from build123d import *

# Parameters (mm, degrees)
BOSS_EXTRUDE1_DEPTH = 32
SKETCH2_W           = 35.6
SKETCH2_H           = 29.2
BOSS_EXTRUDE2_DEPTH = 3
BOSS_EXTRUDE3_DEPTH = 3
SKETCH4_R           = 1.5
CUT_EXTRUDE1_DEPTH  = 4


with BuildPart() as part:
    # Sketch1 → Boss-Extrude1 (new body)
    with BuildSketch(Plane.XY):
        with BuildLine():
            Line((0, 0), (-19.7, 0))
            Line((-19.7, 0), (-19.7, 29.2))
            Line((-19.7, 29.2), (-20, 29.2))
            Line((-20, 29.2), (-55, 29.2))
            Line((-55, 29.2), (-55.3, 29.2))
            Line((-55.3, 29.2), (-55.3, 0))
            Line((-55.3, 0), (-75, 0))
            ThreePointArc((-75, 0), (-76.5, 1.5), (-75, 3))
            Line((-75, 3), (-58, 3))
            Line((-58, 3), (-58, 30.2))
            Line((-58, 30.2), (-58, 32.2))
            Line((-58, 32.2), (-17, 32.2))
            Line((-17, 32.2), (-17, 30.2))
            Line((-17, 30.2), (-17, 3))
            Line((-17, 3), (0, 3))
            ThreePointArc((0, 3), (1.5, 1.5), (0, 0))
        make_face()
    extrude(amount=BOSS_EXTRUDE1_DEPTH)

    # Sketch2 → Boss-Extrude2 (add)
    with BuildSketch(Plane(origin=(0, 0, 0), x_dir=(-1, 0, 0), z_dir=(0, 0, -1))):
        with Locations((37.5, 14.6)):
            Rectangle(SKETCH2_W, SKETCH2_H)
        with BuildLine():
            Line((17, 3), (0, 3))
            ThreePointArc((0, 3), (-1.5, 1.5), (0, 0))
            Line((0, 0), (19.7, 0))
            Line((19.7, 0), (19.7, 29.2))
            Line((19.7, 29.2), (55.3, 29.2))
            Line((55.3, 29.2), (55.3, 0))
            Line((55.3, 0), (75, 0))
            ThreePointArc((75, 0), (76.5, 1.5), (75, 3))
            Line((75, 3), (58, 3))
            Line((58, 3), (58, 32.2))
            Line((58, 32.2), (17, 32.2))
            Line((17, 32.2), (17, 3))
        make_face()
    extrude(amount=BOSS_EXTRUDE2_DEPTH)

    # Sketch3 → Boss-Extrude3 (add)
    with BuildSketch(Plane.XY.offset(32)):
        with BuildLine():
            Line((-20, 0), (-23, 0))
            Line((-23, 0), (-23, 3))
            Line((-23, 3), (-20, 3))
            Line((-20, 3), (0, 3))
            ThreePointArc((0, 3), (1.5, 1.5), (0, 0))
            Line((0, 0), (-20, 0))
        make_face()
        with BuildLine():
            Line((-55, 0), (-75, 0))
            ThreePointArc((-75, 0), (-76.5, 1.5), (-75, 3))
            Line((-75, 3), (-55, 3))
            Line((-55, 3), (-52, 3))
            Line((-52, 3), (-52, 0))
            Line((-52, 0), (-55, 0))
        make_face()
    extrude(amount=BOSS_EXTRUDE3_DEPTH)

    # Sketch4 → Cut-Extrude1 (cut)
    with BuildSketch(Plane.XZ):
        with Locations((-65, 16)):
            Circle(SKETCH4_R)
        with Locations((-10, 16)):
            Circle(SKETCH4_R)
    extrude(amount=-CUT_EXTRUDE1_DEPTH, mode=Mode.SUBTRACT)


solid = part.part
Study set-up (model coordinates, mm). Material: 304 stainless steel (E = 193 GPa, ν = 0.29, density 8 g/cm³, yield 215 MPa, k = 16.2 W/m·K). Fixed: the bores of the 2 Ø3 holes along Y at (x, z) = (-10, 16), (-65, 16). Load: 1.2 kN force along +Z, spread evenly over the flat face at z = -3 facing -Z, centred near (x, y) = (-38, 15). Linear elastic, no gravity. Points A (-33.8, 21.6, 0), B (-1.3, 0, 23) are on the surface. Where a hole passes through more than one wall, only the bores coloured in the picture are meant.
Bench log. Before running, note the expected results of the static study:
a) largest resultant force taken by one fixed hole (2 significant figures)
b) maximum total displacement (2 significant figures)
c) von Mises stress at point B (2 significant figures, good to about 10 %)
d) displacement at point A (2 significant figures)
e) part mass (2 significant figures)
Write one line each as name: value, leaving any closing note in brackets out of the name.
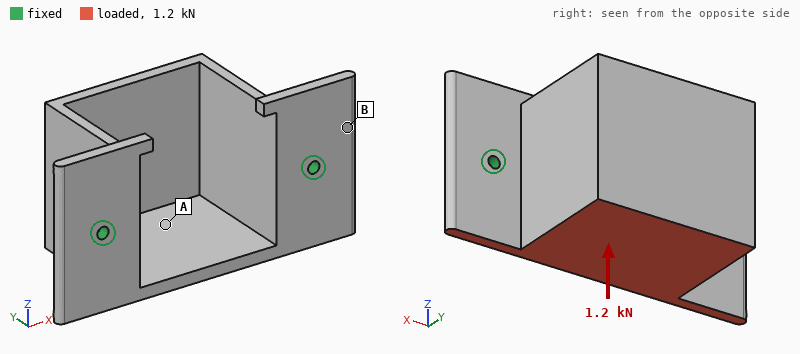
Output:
largest resultant force taken by one fixed hole: 670 N
maximum total displacement: 0.13 mm
von Mises stress at point B: 59 MPa
displacement at point A: 0.100 mm
part mass: 140 g
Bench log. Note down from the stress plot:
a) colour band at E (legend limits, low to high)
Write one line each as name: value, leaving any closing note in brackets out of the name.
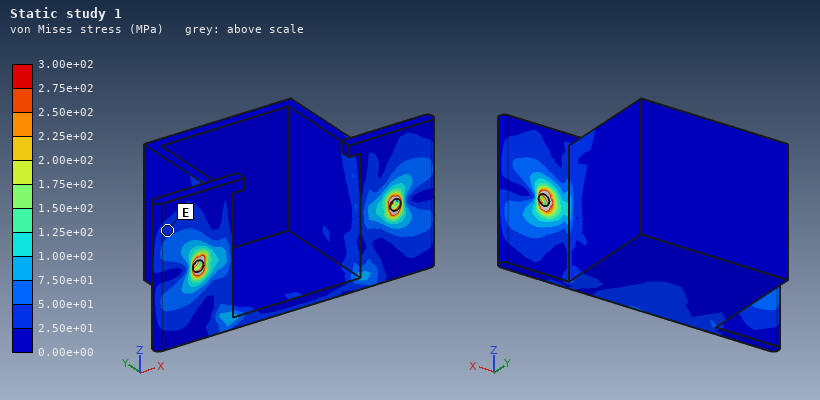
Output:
colour band at E: 2.50e+01 to 5.00e+01 MPa
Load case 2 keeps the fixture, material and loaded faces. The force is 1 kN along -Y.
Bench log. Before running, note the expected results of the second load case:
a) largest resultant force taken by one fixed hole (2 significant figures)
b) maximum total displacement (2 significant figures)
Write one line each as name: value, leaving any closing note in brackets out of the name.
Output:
largest resultant force taken by one fixed hole: 500 N
maximum total displacement: 0.15 mm
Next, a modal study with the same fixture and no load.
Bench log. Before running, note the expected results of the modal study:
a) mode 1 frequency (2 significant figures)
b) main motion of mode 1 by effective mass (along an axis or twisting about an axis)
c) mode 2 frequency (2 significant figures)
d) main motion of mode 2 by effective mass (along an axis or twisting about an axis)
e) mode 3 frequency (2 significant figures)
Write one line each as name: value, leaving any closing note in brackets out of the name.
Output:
mode 1 frequency: 1300 Hz
main motion of mode 1 by effective mass: along Z
mode 2 frequency: 2200 Hz
main motion of mode 2 by effective mass: along X
mode 3 frequency: 5000 Hz
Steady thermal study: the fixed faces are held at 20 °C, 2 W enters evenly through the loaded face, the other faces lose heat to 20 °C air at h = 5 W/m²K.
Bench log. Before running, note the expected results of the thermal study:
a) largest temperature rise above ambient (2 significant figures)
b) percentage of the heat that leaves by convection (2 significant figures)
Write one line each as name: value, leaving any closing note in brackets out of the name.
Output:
largest temperature rise above ambient: 18 K
percentage of the heat that leaves by convection: 27 %
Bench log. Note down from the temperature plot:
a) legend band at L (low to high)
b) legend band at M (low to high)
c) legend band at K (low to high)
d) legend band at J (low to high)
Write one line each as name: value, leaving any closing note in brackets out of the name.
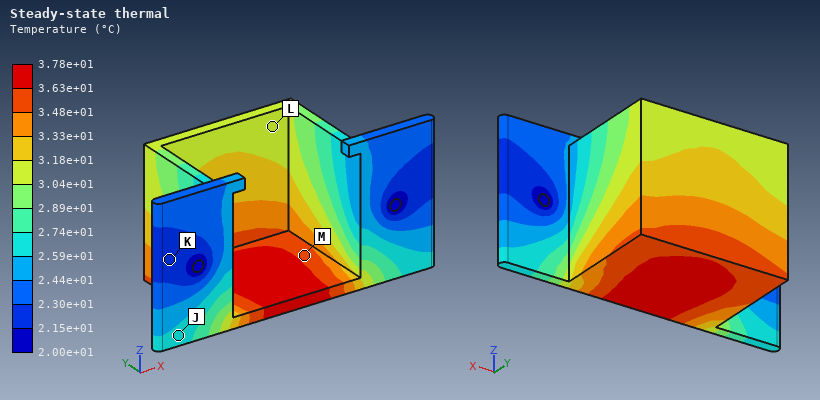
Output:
legend band at L: 3.04e+01 to 3.18e+01 °C
legend band at M: 3.48e+01 to 3.63e+01 °C
legend band at K: 2.15e+01 to 2.30e+01 °C
legend band at J: 2.59e+01 to 2.74e+01 °C
